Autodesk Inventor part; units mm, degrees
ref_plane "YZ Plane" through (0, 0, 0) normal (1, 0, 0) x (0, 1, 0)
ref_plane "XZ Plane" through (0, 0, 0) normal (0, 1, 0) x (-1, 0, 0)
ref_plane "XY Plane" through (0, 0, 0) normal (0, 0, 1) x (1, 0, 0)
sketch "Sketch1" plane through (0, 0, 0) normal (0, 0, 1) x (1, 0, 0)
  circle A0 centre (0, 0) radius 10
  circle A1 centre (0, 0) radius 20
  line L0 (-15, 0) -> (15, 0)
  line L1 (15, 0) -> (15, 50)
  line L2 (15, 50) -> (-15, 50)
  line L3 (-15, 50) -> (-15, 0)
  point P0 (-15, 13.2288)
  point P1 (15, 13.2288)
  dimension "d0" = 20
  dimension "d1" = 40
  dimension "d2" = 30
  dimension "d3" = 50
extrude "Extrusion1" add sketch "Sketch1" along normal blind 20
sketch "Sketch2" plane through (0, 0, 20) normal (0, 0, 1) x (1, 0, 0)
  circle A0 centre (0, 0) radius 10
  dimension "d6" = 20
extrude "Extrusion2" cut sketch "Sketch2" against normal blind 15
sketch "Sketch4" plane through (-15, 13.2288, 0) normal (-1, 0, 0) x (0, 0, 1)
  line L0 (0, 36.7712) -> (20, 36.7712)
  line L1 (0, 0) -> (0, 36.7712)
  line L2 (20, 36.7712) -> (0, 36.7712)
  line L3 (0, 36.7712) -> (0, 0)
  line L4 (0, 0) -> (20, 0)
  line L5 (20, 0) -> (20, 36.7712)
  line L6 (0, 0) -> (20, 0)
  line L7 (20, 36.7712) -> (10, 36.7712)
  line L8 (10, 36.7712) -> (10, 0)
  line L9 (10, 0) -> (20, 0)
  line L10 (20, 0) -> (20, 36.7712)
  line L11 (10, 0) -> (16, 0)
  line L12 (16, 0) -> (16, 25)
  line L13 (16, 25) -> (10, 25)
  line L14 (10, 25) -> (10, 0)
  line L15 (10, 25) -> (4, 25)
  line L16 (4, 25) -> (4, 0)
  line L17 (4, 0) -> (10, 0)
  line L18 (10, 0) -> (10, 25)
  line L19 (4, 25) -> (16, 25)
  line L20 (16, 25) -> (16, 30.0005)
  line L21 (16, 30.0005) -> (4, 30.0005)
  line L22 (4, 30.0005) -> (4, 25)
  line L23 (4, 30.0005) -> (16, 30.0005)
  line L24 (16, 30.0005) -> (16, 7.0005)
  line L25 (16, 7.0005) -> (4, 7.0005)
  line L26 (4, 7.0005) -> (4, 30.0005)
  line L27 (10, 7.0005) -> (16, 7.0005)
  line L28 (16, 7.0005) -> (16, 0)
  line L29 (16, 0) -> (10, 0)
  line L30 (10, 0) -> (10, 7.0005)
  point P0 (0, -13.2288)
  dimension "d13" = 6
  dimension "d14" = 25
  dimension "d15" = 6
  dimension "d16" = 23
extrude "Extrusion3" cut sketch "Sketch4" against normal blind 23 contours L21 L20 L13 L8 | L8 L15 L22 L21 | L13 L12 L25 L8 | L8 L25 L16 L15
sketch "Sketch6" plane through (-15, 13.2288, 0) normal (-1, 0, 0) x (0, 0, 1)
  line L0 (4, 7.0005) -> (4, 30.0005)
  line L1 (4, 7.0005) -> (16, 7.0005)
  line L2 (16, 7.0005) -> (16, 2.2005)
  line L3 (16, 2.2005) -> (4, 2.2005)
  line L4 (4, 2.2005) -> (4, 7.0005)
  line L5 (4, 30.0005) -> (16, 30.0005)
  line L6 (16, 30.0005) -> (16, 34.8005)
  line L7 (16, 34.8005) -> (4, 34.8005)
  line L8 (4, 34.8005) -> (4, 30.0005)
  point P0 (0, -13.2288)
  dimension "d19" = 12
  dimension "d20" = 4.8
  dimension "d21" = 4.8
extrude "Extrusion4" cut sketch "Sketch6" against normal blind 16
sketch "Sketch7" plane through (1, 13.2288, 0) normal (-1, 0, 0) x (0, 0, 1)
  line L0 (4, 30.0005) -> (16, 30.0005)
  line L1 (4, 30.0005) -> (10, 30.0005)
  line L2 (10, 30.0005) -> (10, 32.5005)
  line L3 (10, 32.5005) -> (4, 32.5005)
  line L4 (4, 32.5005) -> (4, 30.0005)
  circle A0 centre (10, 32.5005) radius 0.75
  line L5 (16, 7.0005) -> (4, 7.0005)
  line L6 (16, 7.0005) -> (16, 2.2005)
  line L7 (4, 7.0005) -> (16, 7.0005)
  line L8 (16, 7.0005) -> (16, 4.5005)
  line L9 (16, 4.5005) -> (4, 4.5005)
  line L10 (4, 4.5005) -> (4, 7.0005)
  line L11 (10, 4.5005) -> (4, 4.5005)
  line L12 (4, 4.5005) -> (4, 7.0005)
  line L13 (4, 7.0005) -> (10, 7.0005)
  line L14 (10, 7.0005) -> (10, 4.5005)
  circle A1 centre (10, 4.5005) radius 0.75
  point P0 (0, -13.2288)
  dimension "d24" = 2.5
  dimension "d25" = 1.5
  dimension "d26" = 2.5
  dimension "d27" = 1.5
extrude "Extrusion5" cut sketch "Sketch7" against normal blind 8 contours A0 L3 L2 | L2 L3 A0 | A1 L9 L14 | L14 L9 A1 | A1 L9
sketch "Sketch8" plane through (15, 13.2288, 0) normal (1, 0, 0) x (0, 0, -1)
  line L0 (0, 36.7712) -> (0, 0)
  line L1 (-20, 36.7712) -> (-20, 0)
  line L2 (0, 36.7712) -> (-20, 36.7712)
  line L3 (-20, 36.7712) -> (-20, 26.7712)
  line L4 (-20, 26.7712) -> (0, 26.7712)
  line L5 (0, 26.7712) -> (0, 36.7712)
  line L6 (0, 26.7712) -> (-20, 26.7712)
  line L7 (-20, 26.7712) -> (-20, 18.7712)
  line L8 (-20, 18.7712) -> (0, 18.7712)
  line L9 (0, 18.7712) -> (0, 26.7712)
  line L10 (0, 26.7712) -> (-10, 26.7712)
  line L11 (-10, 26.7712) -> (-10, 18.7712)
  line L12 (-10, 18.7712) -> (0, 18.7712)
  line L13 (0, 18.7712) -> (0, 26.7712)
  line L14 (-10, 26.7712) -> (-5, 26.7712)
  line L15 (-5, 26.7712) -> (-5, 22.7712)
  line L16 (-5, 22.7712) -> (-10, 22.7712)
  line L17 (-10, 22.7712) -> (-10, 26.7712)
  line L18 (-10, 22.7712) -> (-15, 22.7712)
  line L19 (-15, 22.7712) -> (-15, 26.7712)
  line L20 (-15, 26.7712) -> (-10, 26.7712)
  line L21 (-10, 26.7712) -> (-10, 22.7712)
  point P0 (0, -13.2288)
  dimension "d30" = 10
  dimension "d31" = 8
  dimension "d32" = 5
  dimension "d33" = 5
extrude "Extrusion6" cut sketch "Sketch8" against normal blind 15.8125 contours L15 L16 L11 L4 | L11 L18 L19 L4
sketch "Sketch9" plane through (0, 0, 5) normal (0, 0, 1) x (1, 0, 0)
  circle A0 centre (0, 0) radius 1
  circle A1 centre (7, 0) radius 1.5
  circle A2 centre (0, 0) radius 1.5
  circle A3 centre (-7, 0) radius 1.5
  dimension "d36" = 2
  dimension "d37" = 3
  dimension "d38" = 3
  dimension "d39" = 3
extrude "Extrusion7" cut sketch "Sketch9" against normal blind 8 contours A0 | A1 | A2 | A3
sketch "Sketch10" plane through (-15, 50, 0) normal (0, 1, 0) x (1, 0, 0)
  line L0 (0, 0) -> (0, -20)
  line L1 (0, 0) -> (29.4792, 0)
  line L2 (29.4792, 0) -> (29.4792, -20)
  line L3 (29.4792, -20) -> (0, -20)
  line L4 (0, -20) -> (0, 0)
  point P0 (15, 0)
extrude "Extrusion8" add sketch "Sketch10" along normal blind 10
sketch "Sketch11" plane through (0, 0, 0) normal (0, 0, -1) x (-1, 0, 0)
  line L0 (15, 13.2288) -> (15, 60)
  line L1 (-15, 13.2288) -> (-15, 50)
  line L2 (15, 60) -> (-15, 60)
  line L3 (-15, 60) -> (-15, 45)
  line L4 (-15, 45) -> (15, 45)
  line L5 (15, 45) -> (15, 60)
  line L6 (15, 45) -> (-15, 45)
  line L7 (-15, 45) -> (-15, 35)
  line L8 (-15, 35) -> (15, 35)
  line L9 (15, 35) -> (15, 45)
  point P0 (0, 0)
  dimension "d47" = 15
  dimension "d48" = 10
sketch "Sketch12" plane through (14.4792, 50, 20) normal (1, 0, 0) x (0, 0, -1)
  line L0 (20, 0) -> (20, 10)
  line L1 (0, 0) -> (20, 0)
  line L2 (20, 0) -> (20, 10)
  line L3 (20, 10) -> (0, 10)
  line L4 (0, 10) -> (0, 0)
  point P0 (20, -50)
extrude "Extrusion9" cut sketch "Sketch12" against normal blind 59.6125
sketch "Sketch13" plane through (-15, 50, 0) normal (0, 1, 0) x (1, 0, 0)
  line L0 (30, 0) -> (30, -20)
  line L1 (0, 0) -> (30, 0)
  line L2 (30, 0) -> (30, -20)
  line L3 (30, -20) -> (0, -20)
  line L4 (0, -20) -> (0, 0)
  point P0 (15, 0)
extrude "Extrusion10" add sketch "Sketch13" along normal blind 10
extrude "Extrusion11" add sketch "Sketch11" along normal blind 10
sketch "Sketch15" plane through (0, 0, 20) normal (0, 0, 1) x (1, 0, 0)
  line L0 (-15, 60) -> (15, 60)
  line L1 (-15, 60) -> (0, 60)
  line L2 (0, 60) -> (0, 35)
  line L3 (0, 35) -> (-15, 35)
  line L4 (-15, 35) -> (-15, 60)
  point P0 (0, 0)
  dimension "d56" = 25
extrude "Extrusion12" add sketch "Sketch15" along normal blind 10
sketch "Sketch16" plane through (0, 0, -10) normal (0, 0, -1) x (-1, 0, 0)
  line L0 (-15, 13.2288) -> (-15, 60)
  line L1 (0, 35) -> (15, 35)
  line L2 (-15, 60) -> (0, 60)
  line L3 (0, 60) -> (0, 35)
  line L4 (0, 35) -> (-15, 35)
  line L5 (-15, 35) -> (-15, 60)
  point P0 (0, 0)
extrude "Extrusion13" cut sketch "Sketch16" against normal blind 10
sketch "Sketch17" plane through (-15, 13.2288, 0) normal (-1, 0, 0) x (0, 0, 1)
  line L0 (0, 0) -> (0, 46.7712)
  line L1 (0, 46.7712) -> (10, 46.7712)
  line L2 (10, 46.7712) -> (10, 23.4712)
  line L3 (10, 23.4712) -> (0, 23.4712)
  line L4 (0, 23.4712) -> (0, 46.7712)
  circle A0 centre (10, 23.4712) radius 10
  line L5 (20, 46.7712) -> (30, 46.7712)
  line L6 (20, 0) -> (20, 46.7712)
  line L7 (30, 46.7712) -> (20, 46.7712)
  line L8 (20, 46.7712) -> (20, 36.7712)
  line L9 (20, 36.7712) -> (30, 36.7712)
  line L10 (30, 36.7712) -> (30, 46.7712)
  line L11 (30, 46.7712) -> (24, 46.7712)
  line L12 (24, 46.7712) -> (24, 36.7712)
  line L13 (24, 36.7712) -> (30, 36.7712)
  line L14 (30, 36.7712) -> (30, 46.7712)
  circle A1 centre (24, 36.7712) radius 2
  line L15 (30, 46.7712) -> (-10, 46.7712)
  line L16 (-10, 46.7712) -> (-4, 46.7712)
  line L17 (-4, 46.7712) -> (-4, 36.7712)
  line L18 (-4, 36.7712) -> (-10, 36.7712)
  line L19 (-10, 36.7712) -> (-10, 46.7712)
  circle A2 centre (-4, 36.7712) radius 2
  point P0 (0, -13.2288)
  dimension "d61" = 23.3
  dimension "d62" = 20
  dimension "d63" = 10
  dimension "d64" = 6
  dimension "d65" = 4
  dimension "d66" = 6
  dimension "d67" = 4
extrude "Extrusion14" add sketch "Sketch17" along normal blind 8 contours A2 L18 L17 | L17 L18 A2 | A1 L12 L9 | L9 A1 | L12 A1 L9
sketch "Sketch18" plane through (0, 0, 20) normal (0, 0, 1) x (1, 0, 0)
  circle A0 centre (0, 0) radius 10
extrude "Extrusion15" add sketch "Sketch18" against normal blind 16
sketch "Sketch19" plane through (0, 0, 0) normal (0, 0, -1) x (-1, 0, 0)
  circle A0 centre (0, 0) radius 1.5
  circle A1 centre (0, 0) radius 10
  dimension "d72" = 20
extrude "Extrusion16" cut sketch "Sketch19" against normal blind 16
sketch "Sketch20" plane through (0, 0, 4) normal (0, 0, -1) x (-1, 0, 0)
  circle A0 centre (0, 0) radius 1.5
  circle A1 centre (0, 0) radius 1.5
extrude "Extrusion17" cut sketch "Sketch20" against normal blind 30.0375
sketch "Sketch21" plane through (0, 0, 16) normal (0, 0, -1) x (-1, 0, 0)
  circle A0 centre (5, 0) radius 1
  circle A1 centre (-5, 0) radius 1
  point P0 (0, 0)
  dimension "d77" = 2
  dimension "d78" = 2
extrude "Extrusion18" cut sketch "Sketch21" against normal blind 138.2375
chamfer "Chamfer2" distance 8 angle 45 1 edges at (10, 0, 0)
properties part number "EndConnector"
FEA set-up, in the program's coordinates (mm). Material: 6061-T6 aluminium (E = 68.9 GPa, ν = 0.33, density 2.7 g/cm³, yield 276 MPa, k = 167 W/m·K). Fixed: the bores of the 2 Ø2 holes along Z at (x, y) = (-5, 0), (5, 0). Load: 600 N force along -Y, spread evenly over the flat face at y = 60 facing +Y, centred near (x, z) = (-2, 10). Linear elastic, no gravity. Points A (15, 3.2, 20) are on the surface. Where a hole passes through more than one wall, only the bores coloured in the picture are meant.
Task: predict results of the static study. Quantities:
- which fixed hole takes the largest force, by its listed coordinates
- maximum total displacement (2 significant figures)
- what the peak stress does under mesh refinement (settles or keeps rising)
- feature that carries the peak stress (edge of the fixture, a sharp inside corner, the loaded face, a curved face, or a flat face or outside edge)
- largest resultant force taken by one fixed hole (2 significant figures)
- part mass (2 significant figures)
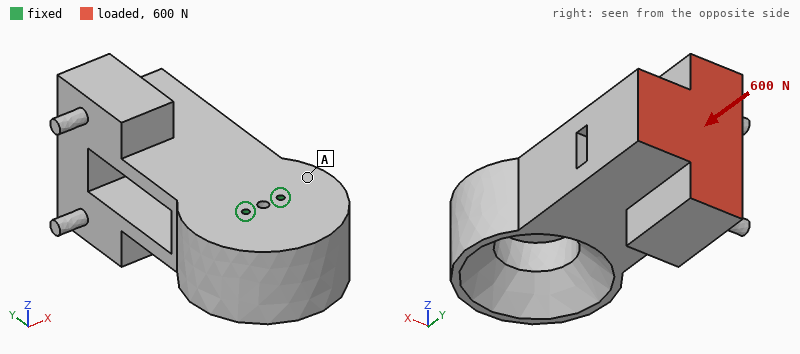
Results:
(-5, 0)
0.11 mm
keeps rising
edge of the fixture
440 N
110 g
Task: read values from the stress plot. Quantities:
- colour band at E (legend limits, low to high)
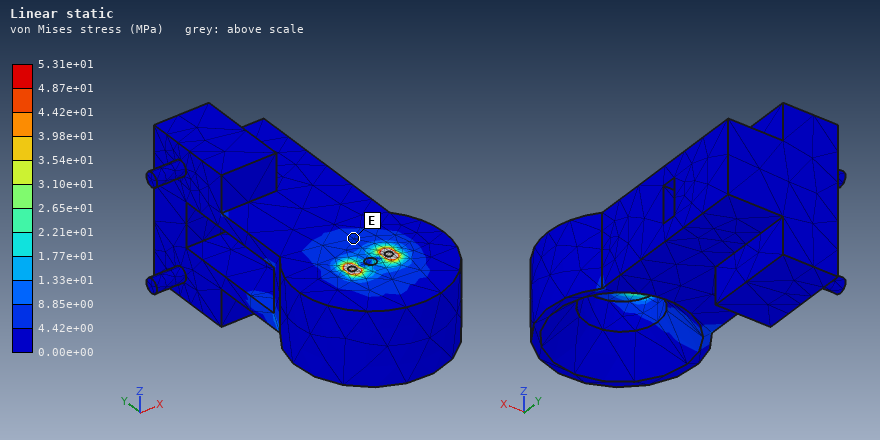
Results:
4.42e+00 to 8.85e+00 MPa
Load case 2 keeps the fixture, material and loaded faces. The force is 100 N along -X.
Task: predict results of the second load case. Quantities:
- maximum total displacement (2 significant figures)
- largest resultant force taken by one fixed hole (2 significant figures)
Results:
22 µm
540 N
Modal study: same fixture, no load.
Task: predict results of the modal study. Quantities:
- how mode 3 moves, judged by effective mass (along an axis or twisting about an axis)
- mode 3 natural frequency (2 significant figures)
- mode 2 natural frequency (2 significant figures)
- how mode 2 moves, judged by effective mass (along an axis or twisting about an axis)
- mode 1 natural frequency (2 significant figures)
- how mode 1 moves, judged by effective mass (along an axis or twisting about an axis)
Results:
twisting about Y
3100 Hz
1800 Hz
along X
680 Hz
along Z
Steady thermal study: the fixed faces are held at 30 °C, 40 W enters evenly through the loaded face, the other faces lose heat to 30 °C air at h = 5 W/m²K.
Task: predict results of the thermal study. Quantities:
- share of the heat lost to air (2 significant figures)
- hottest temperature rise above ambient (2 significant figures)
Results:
4.4 %
46 K
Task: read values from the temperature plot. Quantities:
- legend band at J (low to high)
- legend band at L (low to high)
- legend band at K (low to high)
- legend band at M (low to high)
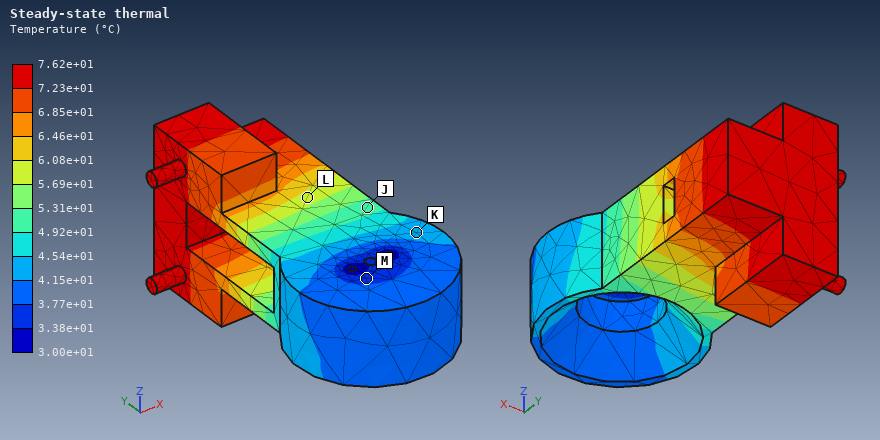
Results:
4.92e+01 to 5.31e+01 °C
5.69e+01 to 6.08e+01 °C
4.15e+01 to 4.54e+01 °C
3.38e+01 to 3.77e+01 °C
